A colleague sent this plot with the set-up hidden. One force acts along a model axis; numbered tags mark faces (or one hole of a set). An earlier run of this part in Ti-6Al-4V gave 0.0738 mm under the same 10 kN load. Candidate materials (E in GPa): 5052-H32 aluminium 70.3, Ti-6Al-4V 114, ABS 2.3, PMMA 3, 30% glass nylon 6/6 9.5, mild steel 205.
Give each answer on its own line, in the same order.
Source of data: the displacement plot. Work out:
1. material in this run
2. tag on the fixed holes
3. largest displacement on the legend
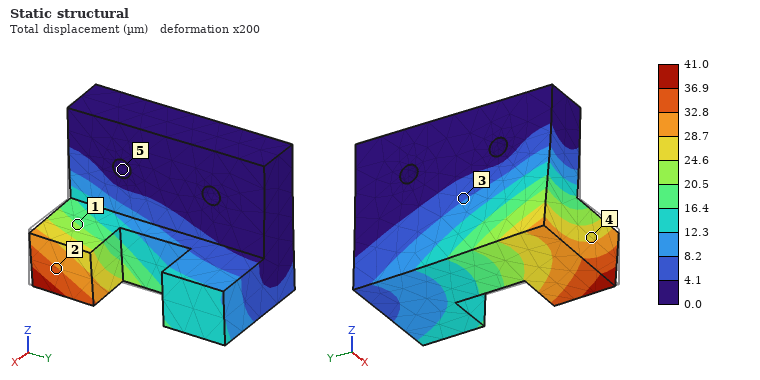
mild steel
5
41.0 µm
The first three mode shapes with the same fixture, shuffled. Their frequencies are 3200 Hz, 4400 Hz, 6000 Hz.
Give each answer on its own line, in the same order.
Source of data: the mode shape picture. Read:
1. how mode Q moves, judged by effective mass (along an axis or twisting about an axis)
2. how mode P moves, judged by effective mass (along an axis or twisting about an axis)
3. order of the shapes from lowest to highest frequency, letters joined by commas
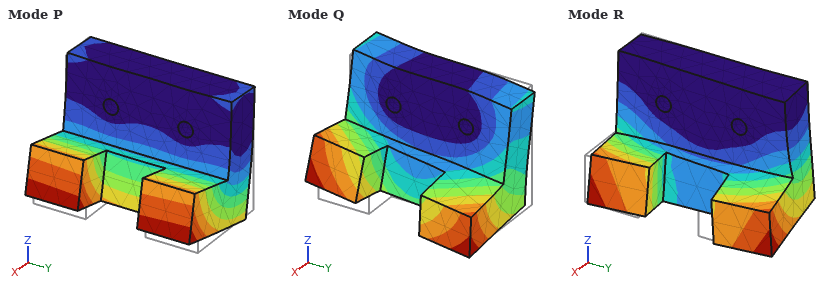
along Y
along X
P, R, Q
